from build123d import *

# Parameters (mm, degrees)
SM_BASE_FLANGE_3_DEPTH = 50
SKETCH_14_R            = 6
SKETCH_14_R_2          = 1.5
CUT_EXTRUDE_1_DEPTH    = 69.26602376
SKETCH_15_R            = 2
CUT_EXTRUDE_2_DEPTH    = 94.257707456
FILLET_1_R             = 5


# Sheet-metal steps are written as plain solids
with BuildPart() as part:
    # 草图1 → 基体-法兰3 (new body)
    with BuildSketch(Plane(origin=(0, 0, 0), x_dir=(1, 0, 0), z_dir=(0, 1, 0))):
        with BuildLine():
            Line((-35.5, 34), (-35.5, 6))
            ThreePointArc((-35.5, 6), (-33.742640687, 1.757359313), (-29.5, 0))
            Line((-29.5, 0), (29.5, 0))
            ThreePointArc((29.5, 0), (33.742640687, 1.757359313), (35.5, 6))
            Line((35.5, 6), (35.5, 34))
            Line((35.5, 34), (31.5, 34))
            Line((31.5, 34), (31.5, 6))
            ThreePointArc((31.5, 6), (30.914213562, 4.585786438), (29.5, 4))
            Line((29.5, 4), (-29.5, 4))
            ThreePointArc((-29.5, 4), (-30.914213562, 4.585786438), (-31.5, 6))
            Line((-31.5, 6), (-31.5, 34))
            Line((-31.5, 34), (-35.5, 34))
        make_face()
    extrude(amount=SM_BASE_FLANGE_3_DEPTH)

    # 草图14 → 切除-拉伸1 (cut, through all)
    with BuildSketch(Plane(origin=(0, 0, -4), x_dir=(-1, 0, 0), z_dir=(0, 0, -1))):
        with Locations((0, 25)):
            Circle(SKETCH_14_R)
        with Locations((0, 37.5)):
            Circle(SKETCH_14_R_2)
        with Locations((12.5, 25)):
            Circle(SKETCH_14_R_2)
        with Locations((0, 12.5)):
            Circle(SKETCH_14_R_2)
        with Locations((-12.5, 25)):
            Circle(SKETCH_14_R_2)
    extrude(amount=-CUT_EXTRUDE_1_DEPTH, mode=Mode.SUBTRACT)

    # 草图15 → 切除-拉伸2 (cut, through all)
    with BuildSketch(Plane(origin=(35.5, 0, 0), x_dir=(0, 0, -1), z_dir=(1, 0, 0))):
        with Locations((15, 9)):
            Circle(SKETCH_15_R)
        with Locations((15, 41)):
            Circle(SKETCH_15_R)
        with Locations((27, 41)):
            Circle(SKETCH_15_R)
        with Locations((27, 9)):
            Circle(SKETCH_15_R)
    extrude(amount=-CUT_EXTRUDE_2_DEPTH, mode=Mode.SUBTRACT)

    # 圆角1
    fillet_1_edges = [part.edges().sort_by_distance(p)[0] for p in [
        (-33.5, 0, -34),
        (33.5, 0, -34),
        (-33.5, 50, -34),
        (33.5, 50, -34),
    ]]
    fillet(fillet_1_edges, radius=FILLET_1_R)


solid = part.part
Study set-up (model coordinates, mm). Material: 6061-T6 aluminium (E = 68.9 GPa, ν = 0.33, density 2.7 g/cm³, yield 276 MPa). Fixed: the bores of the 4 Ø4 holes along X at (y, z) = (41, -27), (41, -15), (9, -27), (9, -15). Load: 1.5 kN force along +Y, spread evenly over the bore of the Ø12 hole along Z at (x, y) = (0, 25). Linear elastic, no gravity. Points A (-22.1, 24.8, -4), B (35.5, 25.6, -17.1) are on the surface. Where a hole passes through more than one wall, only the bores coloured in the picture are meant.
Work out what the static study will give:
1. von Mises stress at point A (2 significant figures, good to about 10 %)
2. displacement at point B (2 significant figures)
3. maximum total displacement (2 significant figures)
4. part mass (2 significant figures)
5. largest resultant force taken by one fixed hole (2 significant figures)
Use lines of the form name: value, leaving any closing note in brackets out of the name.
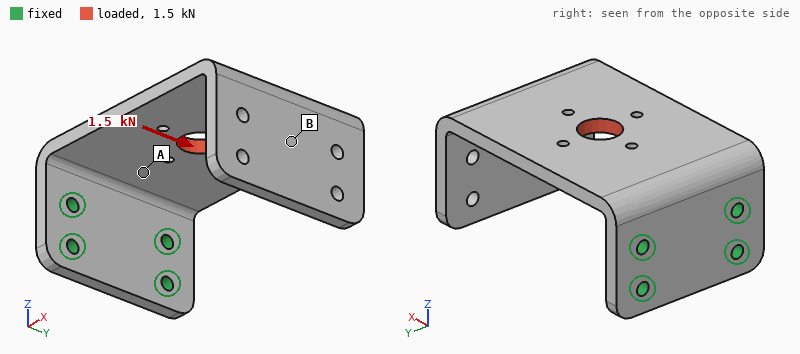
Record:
von Mises stress at point A: 55 MPa
displacement at point B: 0.45 mm
maximum total displacement: 0.57 mm
part mass: 66 g
largest resultant force taken by one fixed hole: 1.9 kN
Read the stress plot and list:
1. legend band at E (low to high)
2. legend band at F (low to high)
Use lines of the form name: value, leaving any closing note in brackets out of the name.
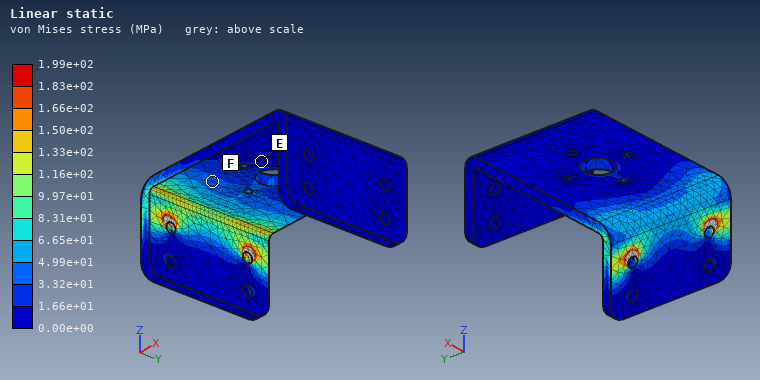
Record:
legend band at E: 0.00e+00 to 1.66e+01 MPa
legend band at F: 3.32e+01 to 4.99e+01 MPa
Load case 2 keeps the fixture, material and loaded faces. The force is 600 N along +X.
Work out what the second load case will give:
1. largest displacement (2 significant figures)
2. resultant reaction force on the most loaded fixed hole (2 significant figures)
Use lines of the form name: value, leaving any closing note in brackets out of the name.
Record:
largest displacement: 0.21 mm
resultant reaction force on the most loaded fixed hole: 400 N
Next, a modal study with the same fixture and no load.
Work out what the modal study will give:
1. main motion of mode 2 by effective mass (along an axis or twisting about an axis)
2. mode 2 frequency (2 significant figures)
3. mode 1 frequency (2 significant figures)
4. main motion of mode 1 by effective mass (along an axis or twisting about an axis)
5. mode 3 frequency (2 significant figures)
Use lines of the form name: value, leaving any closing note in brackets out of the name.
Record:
main motion of mode 2 by effective mass: along Y
mode 2 frequency: 830 Hz
mode 1 frequency: 340 Hz
main motion of mode 1 by effective mass: along Z
mode 3 frequency: 1500 Hz
